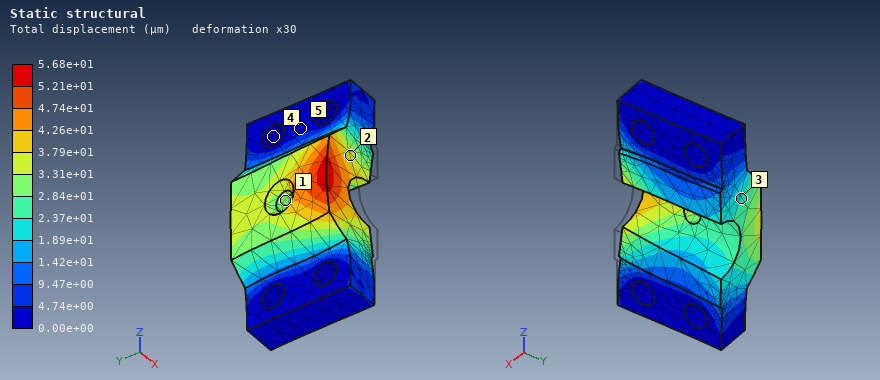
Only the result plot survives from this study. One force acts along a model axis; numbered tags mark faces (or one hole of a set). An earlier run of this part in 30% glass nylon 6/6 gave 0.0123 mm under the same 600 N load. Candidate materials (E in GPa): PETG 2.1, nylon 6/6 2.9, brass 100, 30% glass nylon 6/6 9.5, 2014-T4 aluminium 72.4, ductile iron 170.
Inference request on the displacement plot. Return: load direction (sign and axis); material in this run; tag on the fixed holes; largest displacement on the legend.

+Y
PETG
4
5.68e+01 µm
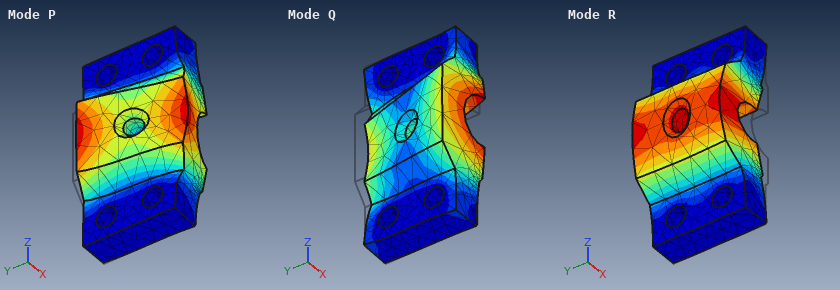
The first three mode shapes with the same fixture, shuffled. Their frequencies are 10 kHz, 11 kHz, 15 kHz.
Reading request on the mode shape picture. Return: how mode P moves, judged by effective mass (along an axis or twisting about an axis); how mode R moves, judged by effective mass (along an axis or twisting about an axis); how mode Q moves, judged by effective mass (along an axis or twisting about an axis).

along Y
along X
along Y
